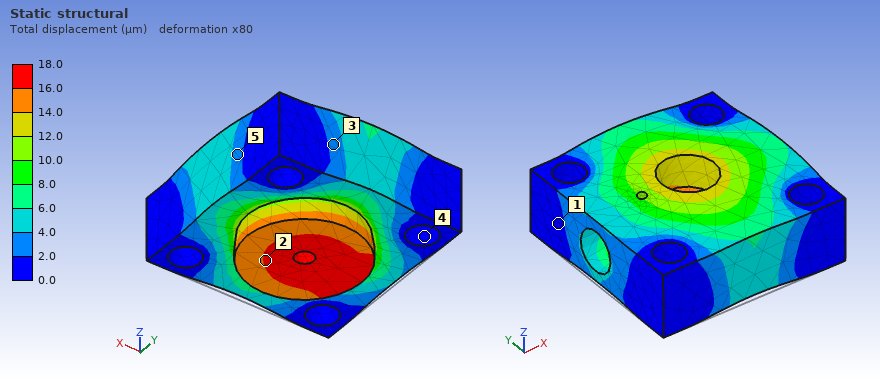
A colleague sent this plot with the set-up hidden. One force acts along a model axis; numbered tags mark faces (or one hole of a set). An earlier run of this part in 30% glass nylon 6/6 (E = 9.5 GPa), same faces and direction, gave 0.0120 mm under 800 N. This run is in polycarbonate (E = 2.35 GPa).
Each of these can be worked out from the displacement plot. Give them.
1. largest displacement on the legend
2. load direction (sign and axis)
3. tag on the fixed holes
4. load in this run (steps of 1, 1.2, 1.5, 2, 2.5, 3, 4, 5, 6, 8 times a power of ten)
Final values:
18.0 µm
+Z
4
300 N
